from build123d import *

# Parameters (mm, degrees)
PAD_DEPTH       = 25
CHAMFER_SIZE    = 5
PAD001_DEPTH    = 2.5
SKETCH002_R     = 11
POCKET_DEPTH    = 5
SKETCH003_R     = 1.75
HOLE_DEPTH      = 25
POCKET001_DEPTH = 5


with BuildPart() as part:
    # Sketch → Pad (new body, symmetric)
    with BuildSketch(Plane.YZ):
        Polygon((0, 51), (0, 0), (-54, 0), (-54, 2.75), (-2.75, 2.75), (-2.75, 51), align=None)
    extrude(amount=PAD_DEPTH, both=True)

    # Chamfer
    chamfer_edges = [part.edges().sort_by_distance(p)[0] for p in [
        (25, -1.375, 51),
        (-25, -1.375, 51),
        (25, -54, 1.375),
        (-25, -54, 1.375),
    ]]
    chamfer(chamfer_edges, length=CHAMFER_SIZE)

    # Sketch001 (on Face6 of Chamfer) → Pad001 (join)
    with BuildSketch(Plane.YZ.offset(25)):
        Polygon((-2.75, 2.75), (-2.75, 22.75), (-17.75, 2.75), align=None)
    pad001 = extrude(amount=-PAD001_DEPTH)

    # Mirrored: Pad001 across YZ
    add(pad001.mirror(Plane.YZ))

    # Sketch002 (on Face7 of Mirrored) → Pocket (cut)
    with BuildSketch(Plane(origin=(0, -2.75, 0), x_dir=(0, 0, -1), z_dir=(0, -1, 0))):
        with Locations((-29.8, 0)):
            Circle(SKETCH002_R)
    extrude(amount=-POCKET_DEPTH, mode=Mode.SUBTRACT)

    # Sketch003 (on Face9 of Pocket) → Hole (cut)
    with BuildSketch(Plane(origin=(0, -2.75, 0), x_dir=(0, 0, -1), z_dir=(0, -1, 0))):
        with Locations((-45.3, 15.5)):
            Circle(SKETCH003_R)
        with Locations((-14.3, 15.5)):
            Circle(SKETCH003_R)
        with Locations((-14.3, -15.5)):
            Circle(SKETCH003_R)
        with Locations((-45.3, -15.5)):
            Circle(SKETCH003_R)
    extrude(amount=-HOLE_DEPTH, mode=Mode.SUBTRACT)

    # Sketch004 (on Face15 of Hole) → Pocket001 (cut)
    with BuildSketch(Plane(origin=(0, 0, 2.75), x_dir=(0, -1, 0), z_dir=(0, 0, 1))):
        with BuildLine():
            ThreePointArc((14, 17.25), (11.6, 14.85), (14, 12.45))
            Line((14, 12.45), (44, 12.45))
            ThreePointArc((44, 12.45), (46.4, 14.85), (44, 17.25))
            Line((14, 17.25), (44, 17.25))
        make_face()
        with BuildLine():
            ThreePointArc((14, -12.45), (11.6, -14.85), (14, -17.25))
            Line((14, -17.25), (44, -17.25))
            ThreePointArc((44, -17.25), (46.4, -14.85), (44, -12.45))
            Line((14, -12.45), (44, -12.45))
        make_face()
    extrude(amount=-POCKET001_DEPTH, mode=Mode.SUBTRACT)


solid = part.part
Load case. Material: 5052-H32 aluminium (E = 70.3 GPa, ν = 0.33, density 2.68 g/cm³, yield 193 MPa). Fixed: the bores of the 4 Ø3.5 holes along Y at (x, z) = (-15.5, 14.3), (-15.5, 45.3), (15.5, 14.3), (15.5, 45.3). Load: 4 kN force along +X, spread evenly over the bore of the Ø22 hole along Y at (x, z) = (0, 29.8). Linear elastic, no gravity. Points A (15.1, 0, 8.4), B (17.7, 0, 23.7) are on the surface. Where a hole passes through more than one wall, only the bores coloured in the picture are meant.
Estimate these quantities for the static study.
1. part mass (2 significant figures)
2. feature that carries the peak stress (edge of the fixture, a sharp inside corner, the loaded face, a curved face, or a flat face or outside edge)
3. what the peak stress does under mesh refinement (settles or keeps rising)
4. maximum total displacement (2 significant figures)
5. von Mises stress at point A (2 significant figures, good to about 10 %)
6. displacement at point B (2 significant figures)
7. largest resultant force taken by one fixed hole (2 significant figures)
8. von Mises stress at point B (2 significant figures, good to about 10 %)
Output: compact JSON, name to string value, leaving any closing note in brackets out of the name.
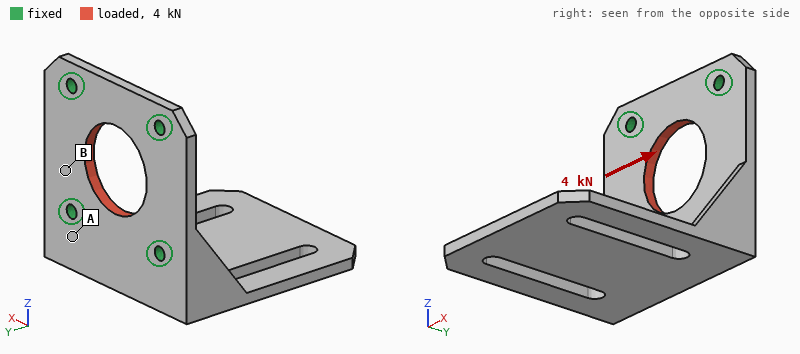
{"part mass": "34 g", "feature that carries the peak stress": "edge of the fixture", "what the peak stress does under mesh refinement": "keeps rising", "maximum total displacement": "9.8 µm", "von Mises stress at point A": "6.2 MPa", "displacement at point B": "6.4 µm", "largest resultant force taken by one fixed hole": "1.0 kN", "von Mises stress at point B": "21 MPa"}
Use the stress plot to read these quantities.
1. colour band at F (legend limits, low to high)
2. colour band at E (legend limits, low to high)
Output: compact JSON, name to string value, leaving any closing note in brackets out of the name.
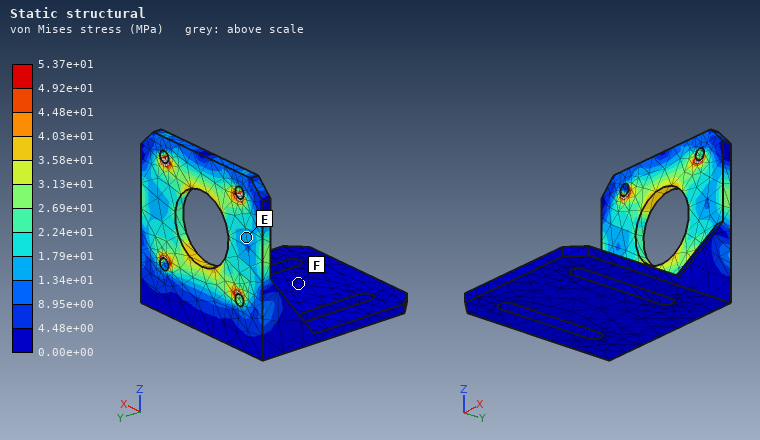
{"colour band at F": "0.00e+00 to 4.48e+00 MPa", "colour band at E": "1.34e+01 to 1.79e+01 MPa"}
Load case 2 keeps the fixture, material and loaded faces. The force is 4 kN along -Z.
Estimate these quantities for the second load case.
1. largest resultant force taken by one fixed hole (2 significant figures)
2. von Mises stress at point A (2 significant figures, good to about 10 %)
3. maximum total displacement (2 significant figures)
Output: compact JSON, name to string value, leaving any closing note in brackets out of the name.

{"largest resultant force taken by one fixed hole": "1.0 kN", "von Mises stress at point A": "14 MPa", "maximum total displacement": "13 µm"}
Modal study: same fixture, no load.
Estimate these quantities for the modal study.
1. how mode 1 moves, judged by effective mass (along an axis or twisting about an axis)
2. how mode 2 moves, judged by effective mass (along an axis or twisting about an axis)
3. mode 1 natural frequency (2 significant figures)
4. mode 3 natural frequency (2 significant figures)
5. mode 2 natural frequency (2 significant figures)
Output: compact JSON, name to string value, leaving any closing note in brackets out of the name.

{"how mode 1 moves, judged by effective mass": "along Z", "how mode 2 moves, judged by effective mass": "along X", "mode 1 natural frequency": "890 Hz", "mode 3 natural frequency": "3100 Hz", "mode 2 natural frequency": "2000 Hz"}
